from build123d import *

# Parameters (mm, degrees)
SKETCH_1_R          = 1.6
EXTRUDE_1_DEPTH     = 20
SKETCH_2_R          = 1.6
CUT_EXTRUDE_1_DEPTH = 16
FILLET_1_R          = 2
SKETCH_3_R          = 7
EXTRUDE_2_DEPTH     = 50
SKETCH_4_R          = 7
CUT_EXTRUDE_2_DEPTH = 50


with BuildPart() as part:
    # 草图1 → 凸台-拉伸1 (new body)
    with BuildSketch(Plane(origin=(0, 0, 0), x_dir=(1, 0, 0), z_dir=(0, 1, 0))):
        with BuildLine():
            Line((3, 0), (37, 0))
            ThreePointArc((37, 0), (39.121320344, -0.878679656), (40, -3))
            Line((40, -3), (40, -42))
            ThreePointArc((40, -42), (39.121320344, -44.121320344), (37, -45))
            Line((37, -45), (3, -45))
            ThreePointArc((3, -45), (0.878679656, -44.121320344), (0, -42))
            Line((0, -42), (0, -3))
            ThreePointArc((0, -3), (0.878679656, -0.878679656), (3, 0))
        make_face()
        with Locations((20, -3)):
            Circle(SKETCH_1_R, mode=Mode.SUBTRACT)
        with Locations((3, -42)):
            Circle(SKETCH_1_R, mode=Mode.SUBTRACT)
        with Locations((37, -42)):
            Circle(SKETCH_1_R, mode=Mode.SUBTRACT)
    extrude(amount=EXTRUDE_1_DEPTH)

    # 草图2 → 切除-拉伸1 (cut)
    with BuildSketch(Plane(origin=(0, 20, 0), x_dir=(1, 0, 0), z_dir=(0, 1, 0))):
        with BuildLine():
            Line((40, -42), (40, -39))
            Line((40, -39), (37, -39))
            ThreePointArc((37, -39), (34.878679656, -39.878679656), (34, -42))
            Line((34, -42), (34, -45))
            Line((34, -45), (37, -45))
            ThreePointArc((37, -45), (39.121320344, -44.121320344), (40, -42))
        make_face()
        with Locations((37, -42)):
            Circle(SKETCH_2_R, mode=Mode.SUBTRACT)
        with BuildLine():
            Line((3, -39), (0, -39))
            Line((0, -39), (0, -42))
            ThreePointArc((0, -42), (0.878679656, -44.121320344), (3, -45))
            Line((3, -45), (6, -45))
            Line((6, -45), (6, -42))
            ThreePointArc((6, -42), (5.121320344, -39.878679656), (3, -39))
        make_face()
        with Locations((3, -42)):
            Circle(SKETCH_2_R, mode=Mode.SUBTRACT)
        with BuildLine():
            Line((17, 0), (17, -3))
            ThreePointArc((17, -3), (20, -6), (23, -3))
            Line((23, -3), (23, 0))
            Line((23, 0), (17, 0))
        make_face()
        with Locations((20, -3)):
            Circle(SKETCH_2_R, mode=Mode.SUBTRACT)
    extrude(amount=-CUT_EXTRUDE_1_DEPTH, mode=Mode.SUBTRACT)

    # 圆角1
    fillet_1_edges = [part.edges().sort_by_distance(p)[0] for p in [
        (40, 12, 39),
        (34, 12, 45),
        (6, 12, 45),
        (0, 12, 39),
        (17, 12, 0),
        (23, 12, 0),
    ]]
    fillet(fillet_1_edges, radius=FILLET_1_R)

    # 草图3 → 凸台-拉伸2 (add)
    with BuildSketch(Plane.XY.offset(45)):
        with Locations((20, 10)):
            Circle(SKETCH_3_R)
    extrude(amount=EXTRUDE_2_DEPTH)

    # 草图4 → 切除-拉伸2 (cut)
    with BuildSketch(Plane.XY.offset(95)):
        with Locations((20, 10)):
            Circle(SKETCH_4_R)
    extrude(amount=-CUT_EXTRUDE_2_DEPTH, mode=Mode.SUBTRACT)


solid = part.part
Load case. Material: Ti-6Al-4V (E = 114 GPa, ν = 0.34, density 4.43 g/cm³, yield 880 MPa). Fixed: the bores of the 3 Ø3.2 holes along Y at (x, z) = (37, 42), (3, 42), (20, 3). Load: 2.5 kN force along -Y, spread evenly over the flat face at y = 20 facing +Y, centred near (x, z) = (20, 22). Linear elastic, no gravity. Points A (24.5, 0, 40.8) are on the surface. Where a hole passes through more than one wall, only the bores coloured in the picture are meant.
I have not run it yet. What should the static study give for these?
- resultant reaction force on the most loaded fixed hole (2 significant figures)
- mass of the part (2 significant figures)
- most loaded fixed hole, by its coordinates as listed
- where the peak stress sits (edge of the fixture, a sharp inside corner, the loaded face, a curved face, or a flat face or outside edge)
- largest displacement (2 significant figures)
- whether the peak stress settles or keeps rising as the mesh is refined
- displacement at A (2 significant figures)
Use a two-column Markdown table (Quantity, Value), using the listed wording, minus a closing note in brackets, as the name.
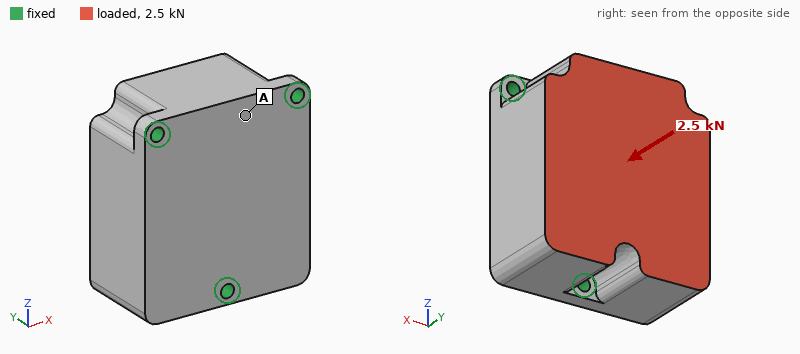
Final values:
| Quantity | Value |
|---|---|
| resultant reaction force on the most loaded fixed hole | 1.3 kN |
| mass of the part | 150 g |
| most loaded fixed hole, by its coordinates as listed | (20, 3) |
| where the peak stress sits | edge of the fixture |
| largest displacement | 3.4 µm |
| whether the peak stress settles or keeps rising as the mesh is refined | keeps rising |
| displacement at A | 2.1 µm |
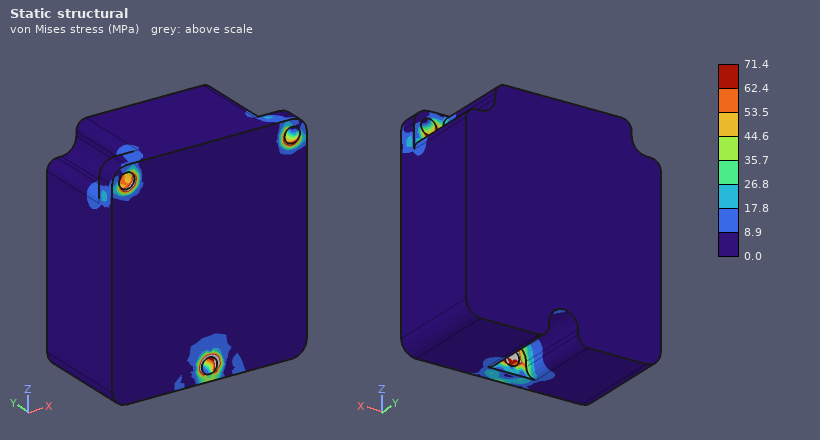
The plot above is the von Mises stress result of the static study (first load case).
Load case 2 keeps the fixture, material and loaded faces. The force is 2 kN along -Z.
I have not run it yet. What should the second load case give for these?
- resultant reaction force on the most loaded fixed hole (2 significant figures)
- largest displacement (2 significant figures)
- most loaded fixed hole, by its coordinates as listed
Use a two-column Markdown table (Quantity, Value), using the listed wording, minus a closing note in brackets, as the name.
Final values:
| Quantity | Value |
|---|---|
| resultant reaction force on the most loaded fixed hole | 1.3 kN |
| largest displacement | 4.2 µm |
| most loaded fixed hole, by its coordinates as listed | (20, 3) |
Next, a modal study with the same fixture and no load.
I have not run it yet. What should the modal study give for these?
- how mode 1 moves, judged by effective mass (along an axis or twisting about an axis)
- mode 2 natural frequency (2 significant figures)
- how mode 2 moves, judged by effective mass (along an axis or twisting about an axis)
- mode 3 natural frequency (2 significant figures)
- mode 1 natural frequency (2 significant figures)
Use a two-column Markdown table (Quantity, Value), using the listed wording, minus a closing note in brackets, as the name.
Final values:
| Quantity | Value |
|---|---|
| how mode 1 moves, judged by effective mass | along X |
| mode 2 natural frequency | 12 kHz |
| how mode 2 moves, judged by effective mass | along Y |
| mode 3 natural frequency | 14 kHz |
| mode 1 natural frequency | 9200 Hz |
